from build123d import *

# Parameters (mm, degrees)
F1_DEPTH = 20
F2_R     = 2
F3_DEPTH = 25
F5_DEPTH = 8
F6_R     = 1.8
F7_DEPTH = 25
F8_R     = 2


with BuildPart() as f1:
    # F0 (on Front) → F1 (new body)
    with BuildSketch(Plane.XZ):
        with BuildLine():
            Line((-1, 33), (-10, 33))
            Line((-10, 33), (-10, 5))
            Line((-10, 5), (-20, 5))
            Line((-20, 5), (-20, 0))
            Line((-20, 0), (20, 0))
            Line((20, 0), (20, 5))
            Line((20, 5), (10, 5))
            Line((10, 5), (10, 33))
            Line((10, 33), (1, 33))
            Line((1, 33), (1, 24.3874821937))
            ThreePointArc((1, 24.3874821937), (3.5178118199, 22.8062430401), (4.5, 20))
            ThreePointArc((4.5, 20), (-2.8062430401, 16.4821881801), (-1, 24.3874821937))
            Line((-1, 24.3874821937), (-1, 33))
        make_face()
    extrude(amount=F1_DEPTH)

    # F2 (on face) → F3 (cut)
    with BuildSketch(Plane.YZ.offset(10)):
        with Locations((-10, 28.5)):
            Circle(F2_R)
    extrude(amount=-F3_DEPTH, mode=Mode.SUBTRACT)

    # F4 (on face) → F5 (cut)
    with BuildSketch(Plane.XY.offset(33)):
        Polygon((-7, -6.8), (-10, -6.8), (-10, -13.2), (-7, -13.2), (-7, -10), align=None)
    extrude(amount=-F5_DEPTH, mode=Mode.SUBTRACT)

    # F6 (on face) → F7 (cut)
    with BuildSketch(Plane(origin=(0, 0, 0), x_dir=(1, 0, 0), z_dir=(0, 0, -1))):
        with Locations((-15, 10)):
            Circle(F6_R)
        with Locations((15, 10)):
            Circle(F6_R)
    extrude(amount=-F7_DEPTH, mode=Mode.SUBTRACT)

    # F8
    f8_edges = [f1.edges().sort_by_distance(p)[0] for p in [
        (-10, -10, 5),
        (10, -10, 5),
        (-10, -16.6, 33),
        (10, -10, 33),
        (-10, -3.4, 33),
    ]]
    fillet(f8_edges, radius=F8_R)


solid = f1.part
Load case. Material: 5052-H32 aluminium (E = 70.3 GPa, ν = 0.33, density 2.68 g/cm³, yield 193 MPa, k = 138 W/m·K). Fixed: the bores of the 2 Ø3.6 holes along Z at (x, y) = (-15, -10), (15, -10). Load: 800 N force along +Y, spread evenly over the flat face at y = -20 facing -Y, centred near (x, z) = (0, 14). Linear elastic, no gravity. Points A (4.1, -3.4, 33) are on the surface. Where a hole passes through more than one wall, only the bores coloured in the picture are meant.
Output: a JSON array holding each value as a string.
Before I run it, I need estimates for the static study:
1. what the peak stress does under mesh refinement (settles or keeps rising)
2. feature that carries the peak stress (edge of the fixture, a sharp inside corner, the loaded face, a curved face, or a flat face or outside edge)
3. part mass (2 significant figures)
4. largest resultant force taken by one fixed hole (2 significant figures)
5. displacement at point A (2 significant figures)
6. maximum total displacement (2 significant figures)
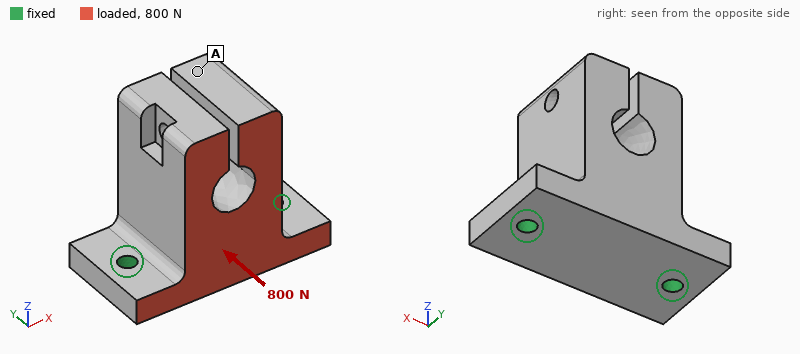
["keeps rising", "edge of the fixture", "35 g", "400 N", "48 µm", "50 µm"]
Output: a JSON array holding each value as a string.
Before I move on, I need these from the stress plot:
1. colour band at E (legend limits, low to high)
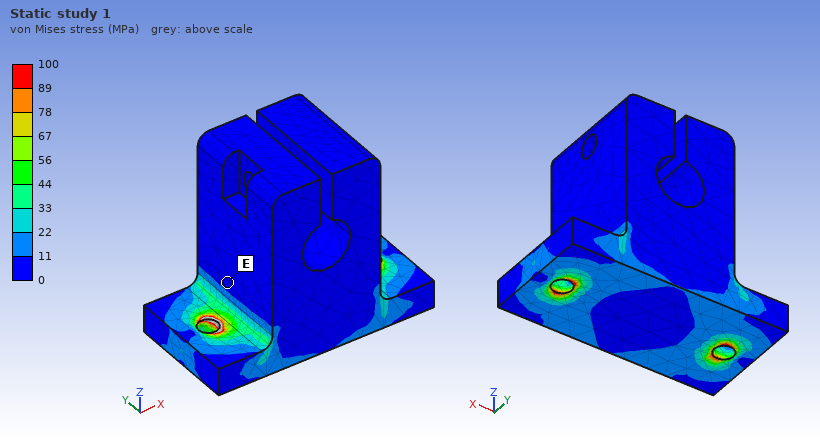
["0 to 11 MPa"]
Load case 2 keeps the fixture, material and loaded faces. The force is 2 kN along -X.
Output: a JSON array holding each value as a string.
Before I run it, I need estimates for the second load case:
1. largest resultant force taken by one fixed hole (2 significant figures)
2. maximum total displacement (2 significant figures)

["1.5 kN", "47 µm"]
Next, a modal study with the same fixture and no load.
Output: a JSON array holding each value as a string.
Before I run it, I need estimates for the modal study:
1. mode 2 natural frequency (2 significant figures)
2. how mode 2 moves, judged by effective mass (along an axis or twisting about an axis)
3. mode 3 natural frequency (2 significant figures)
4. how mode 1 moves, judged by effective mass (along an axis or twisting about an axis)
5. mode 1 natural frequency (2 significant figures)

["8200 Hz", "along X", "10 kHz", "along Y", "4100 Hz"]
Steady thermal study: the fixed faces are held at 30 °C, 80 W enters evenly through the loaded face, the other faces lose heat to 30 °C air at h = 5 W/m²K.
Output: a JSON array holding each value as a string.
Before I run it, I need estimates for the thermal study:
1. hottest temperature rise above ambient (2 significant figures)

["49 K"]
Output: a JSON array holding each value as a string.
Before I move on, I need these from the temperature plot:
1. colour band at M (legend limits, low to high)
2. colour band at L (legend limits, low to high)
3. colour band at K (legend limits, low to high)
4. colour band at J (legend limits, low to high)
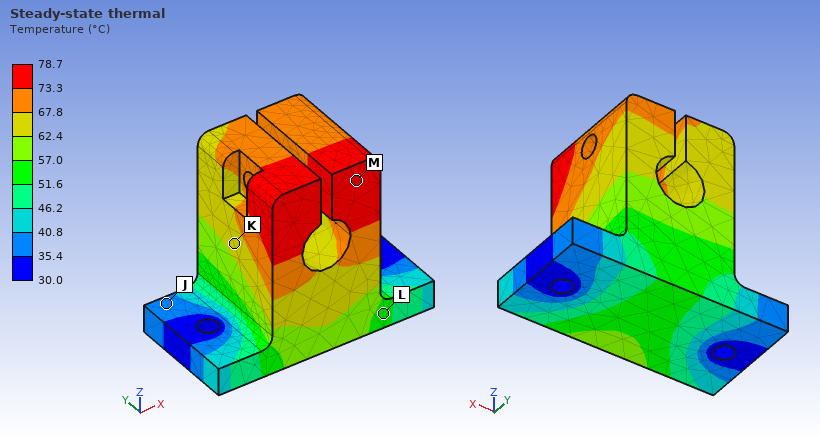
["73.3 to 78.7 °C", "51.6 to 57.0 °C", "62.4 to 67.8 °C", "35.4 to 40.8 °C"]
